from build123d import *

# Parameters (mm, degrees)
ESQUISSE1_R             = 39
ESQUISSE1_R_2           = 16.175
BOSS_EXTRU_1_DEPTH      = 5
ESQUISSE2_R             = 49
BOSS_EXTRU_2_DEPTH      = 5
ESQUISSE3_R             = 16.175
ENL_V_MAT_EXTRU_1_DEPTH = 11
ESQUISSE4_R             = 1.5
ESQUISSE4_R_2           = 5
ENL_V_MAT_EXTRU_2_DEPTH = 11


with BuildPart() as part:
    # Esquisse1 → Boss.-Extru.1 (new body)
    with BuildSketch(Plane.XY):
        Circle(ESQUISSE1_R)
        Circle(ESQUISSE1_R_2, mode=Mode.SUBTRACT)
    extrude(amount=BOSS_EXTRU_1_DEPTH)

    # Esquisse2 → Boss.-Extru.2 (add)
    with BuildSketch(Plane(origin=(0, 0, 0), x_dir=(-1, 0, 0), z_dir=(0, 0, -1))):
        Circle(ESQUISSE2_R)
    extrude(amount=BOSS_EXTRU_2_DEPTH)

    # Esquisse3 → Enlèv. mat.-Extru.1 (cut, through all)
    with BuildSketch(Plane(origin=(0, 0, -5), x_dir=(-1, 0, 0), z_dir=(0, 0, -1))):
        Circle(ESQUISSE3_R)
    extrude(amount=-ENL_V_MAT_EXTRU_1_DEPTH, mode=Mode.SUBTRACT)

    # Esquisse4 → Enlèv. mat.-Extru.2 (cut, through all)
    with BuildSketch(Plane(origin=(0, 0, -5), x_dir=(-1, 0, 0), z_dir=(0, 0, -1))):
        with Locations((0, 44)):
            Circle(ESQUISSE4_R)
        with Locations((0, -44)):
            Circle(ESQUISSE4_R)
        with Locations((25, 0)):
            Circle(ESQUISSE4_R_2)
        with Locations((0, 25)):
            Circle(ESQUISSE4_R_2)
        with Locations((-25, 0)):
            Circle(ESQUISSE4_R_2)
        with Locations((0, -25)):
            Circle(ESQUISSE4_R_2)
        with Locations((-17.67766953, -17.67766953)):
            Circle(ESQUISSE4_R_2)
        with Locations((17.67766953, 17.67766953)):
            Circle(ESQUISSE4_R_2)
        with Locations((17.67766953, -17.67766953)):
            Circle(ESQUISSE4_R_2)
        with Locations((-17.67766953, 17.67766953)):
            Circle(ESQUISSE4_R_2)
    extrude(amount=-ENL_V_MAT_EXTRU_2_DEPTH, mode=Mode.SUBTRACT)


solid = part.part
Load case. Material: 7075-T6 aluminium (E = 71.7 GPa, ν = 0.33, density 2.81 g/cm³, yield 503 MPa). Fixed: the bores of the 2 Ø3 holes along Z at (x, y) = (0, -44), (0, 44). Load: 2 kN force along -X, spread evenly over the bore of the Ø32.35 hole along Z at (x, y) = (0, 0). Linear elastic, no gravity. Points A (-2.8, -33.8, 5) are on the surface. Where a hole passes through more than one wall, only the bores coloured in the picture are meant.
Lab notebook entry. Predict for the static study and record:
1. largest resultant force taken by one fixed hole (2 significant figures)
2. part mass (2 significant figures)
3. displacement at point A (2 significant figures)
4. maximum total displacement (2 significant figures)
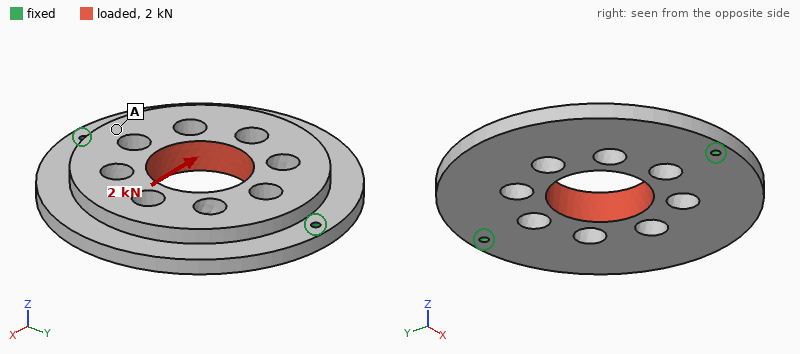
1.0 kN
130 g
9.8 µm
50 µm
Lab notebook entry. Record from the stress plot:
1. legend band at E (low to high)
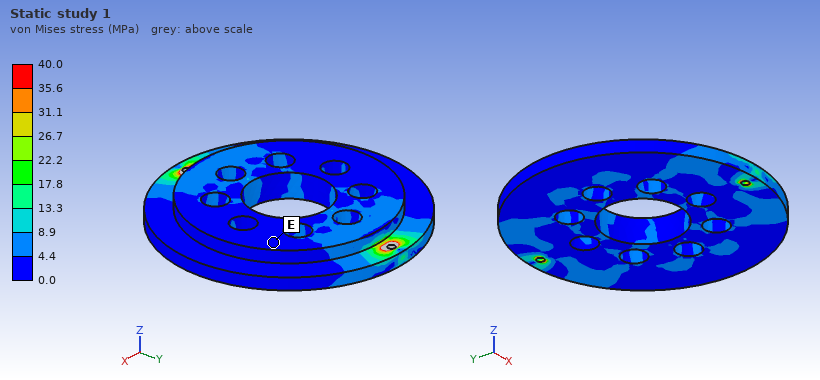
0.0 to 4.4 MPa
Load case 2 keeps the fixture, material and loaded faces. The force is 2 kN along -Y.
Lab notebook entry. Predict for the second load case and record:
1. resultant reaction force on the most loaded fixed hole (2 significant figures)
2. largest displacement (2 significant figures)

1.0 kN
5.5 µm
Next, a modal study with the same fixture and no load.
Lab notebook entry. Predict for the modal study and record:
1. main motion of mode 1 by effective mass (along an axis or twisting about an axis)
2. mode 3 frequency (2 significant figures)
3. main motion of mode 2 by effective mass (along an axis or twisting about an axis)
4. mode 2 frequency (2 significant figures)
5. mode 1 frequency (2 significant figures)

twisting about Y
4900 Hz
along Z
2300 Hz
1200 Hz
